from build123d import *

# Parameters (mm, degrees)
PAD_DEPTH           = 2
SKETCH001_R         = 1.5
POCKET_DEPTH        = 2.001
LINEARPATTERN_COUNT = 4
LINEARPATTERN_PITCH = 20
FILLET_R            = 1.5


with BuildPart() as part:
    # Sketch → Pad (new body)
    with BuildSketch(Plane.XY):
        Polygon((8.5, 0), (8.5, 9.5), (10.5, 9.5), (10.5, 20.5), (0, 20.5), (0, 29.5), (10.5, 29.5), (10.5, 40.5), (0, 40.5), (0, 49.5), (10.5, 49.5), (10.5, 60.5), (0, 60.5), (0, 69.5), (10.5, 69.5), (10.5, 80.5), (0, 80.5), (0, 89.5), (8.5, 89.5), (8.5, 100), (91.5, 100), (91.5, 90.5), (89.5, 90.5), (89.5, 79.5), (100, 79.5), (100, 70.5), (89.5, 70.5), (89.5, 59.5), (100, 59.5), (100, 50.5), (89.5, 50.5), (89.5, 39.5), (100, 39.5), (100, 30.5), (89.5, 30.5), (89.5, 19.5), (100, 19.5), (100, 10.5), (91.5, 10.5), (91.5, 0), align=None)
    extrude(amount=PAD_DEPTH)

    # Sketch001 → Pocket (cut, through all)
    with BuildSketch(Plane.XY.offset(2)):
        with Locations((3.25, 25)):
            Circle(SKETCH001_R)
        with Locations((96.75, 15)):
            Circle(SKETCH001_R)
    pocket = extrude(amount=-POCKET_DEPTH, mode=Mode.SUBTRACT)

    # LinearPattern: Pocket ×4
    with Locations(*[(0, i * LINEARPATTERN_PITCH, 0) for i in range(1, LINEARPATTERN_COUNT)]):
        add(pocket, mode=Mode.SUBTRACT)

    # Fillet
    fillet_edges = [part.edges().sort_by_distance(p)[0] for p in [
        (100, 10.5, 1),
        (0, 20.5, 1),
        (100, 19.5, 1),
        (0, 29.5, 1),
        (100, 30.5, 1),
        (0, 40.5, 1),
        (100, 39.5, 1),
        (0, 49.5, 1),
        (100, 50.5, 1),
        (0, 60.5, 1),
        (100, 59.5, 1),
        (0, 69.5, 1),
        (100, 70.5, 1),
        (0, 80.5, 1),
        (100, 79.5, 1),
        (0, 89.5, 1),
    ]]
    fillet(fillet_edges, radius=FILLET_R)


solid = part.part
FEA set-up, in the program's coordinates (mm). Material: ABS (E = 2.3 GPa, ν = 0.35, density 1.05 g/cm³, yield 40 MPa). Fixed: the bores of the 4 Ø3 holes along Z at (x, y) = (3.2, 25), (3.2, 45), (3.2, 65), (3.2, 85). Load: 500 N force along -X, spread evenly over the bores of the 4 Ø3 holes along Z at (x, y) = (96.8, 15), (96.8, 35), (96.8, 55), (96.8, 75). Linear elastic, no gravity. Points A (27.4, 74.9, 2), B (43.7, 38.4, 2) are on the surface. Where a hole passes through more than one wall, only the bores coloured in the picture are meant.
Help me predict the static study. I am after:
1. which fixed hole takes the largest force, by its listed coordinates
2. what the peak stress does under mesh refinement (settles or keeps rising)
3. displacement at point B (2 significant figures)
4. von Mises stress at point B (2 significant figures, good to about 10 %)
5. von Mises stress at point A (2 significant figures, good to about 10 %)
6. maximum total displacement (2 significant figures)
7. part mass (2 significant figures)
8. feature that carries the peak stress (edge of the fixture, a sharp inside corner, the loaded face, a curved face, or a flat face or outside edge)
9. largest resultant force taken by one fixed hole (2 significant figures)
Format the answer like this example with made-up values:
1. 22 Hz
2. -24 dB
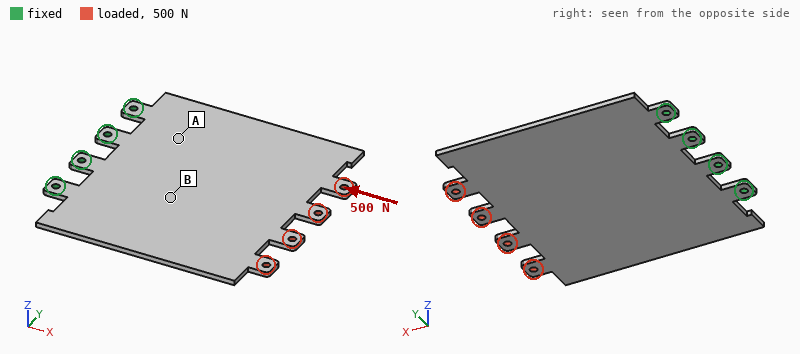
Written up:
1. (3.2, 25)
2. keeps rising
3. 0.11 mm
4. 3.9 MPa
5. 2.0 MPa
6. 0.26 mm
7. 18 g
8. edge of the fixture
9. 210 N
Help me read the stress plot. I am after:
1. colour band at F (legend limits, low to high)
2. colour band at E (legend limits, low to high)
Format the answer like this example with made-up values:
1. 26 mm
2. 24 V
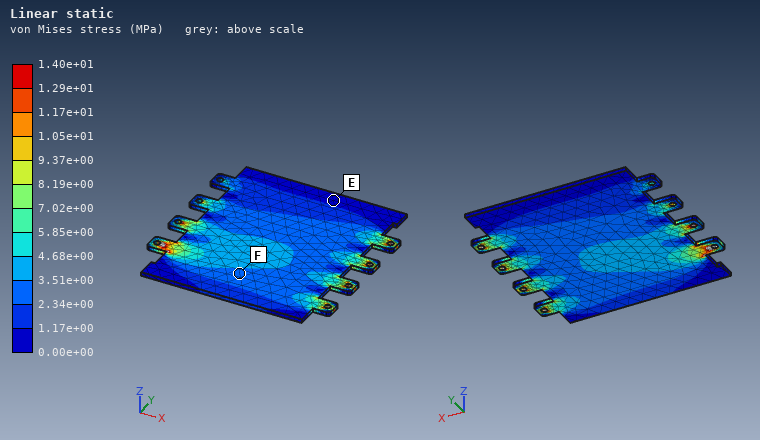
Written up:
1. 2.34e+00 to 3.51e+00 MPa
2. 0.00e+00 to 1.17e+00 MPa
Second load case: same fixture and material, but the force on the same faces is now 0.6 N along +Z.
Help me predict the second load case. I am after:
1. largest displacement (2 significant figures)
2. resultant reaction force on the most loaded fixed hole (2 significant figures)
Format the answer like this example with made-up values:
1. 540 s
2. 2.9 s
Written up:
1. 1.6 mm
2. 0.31 N
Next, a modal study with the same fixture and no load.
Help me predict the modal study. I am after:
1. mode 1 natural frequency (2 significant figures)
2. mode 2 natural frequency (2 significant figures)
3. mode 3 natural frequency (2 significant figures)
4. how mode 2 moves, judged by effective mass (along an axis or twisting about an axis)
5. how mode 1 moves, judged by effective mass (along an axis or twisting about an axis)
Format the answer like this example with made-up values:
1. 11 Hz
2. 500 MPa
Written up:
1. 48 Hz
2. 110 Hz
3. 290 Hz
4. twisting about X
5. along Z
